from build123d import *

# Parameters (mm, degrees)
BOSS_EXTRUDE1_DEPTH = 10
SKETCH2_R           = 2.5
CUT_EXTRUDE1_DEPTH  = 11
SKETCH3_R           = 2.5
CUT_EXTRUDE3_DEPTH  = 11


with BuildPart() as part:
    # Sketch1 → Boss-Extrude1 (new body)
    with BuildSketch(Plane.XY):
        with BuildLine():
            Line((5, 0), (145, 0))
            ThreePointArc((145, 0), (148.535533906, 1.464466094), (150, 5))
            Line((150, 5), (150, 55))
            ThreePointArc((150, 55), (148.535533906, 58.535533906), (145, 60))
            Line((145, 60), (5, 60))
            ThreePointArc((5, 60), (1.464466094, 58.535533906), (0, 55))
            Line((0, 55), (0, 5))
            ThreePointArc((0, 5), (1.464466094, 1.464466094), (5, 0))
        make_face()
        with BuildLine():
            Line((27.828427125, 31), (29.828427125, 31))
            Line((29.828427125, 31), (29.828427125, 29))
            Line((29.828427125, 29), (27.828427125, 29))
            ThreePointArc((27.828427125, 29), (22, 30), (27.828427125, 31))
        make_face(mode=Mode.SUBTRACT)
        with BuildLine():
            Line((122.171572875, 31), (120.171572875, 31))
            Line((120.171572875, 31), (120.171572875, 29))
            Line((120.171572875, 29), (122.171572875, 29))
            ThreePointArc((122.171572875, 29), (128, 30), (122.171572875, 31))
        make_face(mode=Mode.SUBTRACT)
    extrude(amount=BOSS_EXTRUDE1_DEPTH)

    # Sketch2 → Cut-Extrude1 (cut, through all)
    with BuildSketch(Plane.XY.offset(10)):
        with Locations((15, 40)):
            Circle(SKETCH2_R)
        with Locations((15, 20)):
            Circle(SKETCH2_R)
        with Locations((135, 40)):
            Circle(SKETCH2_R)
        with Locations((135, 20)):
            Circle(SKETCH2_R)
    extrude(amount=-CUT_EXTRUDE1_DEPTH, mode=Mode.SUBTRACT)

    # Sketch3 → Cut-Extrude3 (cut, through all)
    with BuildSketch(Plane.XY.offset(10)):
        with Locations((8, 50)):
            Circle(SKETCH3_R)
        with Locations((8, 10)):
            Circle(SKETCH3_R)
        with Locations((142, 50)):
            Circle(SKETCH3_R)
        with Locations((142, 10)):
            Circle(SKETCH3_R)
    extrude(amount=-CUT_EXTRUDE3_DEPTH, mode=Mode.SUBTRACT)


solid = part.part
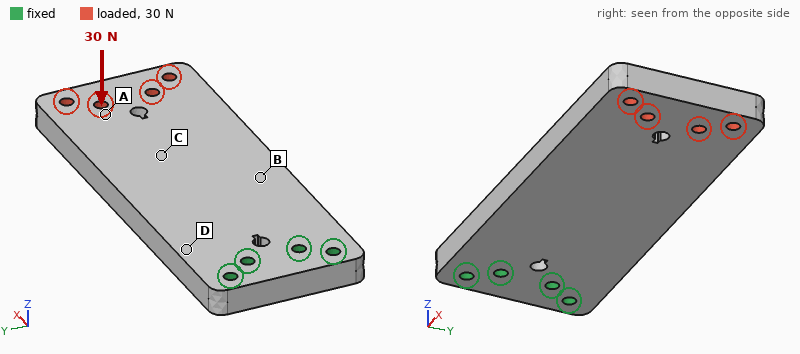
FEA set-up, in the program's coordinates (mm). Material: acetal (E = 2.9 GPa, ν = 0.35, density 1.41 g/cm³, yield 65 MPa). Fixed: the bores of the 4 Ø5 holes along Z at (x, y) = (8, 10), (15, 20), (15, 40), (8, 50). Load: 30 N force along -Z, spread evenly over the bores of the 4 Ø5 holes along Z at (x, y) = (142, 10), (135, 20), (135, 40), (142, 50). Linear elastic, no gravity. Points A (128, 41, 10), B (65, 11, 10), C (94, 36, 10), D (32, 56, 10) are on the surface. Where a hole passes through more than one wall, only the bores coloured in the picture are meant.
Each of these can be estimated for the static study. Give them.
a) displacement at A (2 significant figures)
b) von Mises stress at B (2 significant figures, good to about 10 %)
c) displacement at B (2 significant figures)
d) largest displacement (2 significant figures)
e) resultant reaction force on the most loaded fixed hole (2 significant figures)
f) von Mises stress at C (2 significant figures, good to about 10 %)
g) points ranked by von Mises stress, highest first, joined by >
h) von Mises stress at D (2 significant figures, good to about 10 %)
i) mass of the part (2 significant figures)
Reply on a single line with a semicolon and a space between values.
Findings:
1.2 mm; 2.2 MPa; 0.30 mm; 1.5 mm; 60 N; 1.3 MPa; D > B > C > A; 3.2 MPa; 120 g
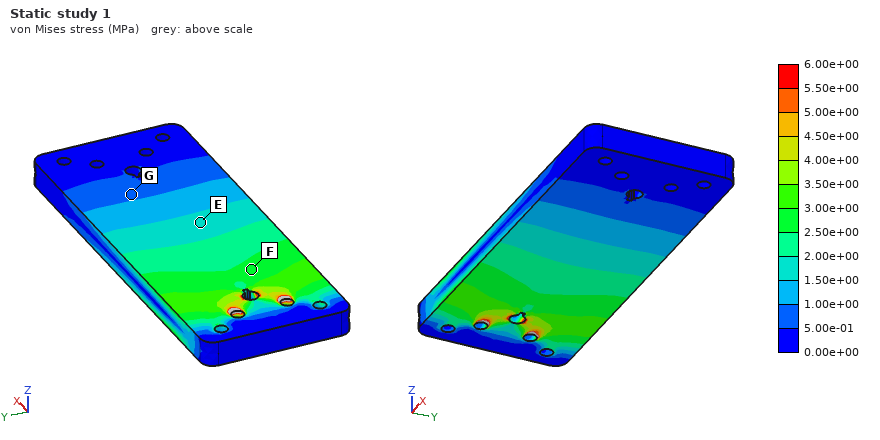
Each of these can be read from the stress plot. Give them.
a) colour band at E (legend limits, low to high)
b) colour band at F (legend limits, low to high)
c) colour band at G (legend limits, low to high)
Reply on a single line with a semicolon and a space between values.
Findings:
1.50e+00 to 2.00e+00 MPa; 2.50e+00 to 3.00e+00 MPa; 5.00e-01 to 1.00e+00 MPa
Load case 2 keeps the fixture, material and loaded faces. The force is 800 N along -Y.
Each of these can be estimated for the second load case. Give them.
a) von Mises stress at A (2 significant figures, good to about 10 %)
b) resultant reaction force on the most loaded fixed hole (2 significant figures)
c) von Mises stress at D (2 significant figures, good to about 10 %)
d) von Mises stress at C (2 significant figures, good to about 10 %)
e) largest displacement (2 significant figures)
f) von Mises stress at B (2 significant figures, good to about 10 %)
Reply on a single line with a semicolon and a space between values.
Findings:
3.5 MPa; 1.8 kN; 12 MPa; 3.6 MPa; 1.6 mm; 6.5 MPa
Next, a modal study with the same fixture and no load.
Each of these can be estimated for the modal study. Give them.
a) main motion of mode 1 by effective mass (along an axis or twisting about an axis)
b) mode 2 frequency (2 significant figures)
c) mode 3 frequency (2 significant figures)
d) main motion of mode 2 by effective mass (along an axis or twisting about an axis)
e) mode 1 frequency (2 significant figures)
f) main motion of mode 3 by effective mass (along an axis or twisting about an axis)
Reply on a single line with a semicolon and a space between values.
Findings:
along Z; 550 Hz; 610 Hz; twisting about X; 130 Hz; along Y
